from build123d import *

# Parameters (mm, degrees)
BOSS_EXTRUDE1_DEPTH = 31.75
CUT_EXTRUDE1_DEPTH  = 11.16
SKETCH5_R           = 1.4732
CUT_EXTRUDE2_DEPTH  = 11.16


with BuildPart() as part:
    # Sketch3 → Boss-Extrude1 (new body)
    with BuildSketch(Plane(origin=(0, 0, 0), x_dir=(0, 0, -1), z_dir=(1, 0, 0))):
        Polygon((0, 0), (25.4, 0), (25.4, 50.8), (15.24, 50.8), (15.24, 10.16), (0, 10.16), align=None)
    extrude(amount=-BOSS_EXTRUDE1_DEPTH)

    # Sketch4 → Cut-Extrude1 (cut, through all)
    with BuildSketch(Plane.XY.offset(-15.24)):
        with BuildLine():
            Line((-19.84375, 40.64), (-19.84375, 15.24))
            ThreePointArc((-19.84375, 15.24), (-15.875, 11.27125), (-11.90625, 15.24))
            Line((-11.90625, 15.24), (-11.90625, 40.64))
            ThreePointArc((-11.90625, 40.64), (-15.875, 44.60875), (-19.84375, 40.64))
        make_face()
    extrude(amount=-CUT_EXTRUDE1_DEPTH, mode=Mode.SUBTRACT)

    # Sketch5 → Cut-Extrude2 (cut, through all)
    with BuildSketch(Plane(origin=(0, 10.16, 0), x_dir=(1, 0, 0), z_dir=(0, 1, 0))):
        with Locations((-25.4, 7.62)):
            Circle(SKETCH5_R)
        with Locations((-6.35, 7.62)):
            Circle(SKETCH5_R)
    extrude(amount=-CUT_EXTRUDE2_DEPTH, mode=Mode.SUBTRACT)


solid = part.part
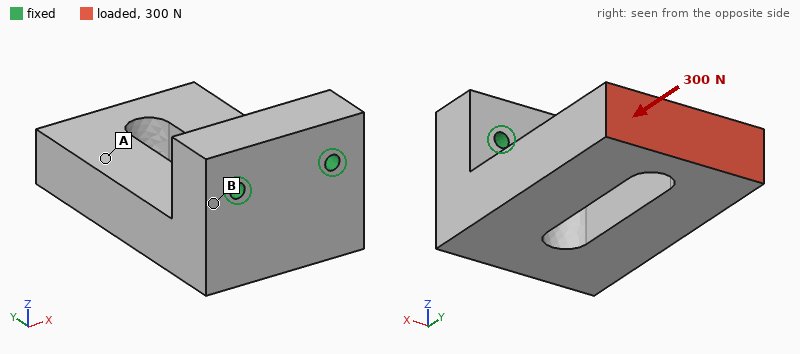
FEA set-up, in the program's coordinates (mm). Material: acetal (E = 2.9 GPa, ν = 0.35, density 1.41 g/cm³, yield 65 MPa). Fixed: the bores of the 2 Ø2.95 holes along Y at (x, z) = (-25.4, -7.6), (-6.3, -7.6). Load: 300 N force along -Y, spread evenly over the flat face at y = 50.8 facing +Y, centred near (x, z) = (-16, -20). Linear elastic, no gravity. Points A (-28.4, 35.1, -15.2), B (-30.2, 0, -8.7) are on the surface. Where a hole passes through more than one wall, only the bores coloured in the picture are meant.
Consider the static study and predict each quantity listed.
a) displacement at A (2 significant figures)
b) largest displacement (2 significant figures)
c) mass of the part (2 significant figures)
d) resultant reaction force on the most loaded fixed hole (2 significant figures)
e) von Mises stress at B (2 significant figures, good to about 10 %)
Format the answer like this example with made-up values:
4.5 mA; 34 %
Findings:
0.13 mm; 0.22 mm; 26 g; 150 N; 3.7 MPa
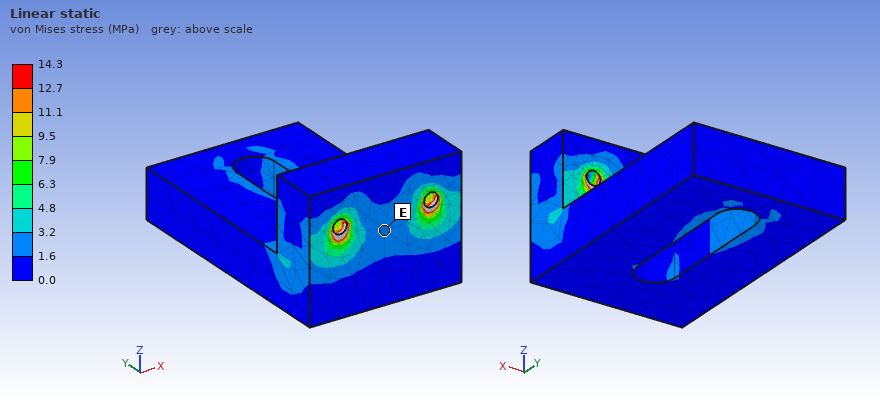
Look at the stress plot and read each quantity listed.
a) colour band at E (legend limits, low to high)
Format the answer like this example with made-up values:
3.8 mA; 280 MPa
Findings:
1.6 to 3.2 MPa
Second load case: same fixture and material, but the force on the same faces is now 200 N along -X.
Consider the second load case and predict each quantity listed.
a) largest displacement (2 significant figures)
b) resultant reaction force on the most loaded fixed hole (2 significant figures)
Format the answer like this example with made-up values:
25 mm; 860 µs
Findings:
0.53 mm; 400 N
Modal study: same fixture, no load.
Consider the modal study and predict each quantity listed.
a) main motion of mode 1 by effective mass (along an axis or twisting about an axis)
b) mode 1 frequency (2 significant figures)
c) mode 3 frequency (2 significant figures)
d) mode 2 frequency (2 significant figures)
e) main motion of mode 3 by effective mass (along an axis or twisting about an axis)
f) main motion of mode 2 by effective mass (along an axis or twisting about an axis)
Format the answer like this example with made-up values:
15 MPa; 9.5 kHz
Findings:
along Z; 790 Hz; 2300 Hz; 1300 Hz; twisting about Y; along X
